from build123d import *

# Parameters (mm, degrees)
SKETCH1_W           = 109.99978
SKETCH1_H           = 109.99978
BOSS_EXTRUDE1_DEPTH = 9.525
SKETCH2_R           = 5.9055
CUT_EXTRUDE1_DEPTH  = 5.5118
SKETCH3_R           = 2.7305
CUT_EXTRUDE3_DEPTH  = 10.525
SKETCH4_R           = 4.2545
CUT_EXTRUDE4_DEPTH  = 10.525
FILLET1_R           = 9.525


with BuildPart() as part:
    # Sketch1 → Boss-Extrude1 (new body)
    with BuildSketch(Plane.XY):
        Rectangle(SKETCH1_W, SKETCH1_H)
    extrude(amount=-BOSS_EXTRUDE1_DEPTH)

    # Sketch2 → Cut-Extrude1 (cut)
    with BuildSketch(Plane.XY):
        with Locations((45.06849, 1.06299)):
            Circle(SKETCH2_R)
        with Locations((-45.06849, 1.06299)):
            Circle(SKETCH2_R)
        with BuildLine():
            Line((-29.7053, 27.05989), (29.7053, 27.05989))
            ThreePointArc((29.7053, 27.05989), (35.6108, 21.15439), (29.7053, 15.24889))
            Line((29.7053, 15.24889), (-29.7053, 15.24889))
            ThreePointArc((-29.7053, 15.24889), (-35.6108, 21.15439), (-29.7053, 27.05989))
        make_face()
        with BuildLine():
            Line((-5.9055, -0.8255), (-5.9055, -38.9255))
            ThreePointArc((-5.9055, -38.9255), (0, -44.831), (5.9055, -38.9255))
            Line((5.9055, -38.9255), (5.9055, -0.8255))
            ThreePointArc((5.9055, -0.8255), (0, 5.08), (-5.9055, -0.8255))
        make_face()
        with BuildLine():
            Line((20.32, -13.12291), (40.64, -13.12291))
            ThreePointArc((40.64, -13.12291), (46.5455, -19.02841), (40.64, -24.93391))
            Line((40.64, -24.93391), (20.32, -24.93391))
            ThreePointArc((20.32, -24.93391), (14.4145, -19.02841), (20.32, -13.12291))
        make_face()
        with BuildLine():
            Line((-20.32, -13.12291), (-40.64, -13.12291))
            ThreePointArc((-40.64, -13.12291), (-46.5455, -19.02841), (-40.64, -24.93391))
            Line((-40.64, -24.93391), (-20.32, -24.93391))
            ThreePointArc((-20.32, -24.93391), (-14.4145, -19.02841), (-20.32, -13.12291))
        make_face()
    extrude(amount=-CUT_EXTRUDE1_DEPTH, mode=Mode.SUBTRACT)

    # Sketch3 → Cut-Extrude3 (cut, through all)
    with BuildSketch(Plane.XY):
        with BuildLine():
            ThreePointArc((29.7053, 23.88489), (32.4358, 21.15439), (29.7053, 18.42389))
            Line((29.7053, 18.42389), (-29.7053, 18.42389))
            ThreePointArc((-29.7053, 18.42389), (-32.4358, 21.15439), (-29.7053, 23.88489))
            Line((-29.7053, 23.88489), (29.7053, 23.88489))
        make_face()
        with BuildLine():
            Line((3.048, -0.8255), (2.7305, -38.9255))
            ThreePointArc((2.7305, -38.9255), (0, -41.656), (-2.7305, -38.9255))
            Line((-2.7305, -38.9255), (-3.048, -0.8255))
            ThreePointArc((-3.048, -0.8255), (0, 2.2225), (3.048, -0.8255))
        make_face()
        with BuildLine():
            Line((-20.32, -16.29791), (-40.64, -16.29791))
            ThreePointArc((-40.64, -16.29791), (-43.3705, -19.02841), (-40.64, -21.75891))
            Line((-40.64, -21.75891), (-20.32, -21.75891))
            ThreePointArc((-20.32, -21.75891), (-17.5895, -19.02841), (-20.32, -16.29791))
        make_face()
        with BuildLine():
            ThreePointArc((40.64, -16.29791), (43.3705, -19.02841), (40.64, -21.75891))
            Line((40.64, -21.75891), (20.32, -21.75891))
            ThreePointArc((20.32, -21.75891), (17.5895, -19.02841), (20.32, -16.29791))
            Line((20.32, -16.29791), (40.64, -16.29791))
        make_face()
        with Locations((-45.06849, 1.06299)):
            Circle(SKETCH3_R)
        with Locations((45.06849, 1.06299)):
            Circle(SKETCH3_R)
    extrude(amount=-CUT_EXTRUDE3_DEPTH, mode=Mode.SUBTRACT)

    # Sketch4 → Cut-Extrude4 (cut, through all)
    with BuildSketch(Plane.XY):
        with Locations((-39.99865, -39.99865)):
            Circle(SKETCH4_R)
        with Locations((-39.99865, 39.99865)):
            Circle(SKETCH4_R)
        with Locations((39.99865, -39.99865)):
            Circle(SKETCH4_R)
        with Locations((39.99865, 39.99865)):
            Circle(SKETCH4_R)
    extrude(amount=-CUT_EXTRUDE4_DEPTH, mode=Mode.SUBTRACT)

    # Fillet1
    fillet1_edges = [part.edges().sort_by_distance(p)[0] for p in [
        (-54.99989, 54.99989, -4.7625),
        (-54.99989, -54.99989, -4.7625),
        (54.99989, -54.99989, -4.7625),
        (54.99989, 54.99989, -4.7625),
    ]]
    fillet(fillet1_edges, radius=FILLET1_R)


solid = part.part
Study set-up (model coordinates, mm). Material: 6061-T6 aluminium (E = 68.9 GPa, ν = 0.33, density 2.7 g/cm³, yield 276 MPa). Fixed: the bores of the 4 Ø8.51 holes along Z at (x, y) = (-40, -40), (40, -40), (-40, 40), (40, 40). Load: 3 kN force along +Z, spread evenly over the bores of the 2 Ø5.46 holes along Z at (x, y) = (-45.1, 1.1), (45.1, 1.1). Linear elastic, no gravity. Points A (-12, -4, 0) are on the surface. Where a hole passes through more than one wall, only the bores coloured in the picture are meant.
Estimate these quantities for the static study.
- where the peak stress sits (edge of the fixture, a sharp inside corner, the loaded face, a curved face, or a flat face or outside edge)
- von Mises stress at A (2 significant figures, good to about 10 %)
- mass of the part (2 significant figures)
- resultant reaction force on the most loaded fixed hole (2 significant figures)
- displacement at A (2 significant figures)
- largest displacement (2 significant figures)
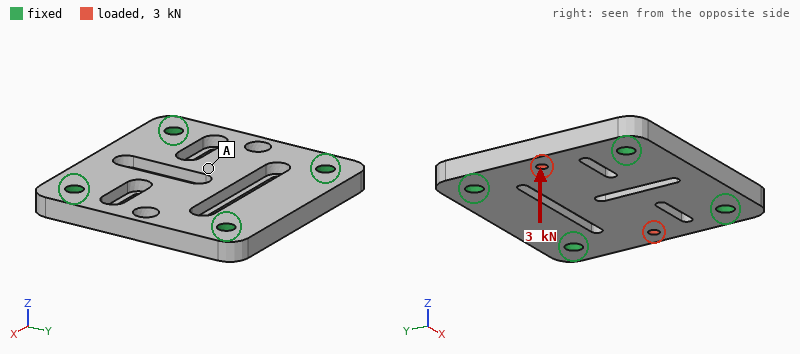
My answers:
the loaded face
8.9 MPa
260 g
820 N
18 µm
48 µm
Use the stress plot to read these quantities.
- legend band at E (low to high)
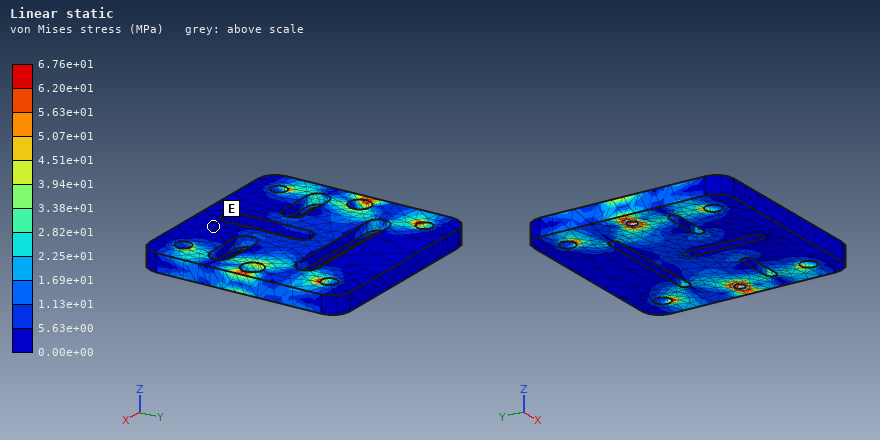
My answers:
0.00e+00 to 5.63e+00 MPa
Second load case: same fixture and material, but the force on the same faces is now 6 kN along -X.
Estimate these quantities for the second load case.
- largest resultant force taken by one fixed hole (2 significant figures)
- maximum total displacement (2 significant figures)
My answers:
1.5 kN
24 µm
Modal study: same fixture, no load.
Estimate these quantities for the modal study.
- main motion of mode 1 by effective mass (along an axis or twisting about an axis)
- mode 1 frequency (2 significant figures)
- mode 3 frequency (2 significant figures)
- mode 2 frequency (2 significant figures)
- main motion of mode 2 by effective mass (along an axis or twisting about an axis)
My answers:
along Z
4100 Hz
7400 Hz
6900 Hz
twisting about Y
